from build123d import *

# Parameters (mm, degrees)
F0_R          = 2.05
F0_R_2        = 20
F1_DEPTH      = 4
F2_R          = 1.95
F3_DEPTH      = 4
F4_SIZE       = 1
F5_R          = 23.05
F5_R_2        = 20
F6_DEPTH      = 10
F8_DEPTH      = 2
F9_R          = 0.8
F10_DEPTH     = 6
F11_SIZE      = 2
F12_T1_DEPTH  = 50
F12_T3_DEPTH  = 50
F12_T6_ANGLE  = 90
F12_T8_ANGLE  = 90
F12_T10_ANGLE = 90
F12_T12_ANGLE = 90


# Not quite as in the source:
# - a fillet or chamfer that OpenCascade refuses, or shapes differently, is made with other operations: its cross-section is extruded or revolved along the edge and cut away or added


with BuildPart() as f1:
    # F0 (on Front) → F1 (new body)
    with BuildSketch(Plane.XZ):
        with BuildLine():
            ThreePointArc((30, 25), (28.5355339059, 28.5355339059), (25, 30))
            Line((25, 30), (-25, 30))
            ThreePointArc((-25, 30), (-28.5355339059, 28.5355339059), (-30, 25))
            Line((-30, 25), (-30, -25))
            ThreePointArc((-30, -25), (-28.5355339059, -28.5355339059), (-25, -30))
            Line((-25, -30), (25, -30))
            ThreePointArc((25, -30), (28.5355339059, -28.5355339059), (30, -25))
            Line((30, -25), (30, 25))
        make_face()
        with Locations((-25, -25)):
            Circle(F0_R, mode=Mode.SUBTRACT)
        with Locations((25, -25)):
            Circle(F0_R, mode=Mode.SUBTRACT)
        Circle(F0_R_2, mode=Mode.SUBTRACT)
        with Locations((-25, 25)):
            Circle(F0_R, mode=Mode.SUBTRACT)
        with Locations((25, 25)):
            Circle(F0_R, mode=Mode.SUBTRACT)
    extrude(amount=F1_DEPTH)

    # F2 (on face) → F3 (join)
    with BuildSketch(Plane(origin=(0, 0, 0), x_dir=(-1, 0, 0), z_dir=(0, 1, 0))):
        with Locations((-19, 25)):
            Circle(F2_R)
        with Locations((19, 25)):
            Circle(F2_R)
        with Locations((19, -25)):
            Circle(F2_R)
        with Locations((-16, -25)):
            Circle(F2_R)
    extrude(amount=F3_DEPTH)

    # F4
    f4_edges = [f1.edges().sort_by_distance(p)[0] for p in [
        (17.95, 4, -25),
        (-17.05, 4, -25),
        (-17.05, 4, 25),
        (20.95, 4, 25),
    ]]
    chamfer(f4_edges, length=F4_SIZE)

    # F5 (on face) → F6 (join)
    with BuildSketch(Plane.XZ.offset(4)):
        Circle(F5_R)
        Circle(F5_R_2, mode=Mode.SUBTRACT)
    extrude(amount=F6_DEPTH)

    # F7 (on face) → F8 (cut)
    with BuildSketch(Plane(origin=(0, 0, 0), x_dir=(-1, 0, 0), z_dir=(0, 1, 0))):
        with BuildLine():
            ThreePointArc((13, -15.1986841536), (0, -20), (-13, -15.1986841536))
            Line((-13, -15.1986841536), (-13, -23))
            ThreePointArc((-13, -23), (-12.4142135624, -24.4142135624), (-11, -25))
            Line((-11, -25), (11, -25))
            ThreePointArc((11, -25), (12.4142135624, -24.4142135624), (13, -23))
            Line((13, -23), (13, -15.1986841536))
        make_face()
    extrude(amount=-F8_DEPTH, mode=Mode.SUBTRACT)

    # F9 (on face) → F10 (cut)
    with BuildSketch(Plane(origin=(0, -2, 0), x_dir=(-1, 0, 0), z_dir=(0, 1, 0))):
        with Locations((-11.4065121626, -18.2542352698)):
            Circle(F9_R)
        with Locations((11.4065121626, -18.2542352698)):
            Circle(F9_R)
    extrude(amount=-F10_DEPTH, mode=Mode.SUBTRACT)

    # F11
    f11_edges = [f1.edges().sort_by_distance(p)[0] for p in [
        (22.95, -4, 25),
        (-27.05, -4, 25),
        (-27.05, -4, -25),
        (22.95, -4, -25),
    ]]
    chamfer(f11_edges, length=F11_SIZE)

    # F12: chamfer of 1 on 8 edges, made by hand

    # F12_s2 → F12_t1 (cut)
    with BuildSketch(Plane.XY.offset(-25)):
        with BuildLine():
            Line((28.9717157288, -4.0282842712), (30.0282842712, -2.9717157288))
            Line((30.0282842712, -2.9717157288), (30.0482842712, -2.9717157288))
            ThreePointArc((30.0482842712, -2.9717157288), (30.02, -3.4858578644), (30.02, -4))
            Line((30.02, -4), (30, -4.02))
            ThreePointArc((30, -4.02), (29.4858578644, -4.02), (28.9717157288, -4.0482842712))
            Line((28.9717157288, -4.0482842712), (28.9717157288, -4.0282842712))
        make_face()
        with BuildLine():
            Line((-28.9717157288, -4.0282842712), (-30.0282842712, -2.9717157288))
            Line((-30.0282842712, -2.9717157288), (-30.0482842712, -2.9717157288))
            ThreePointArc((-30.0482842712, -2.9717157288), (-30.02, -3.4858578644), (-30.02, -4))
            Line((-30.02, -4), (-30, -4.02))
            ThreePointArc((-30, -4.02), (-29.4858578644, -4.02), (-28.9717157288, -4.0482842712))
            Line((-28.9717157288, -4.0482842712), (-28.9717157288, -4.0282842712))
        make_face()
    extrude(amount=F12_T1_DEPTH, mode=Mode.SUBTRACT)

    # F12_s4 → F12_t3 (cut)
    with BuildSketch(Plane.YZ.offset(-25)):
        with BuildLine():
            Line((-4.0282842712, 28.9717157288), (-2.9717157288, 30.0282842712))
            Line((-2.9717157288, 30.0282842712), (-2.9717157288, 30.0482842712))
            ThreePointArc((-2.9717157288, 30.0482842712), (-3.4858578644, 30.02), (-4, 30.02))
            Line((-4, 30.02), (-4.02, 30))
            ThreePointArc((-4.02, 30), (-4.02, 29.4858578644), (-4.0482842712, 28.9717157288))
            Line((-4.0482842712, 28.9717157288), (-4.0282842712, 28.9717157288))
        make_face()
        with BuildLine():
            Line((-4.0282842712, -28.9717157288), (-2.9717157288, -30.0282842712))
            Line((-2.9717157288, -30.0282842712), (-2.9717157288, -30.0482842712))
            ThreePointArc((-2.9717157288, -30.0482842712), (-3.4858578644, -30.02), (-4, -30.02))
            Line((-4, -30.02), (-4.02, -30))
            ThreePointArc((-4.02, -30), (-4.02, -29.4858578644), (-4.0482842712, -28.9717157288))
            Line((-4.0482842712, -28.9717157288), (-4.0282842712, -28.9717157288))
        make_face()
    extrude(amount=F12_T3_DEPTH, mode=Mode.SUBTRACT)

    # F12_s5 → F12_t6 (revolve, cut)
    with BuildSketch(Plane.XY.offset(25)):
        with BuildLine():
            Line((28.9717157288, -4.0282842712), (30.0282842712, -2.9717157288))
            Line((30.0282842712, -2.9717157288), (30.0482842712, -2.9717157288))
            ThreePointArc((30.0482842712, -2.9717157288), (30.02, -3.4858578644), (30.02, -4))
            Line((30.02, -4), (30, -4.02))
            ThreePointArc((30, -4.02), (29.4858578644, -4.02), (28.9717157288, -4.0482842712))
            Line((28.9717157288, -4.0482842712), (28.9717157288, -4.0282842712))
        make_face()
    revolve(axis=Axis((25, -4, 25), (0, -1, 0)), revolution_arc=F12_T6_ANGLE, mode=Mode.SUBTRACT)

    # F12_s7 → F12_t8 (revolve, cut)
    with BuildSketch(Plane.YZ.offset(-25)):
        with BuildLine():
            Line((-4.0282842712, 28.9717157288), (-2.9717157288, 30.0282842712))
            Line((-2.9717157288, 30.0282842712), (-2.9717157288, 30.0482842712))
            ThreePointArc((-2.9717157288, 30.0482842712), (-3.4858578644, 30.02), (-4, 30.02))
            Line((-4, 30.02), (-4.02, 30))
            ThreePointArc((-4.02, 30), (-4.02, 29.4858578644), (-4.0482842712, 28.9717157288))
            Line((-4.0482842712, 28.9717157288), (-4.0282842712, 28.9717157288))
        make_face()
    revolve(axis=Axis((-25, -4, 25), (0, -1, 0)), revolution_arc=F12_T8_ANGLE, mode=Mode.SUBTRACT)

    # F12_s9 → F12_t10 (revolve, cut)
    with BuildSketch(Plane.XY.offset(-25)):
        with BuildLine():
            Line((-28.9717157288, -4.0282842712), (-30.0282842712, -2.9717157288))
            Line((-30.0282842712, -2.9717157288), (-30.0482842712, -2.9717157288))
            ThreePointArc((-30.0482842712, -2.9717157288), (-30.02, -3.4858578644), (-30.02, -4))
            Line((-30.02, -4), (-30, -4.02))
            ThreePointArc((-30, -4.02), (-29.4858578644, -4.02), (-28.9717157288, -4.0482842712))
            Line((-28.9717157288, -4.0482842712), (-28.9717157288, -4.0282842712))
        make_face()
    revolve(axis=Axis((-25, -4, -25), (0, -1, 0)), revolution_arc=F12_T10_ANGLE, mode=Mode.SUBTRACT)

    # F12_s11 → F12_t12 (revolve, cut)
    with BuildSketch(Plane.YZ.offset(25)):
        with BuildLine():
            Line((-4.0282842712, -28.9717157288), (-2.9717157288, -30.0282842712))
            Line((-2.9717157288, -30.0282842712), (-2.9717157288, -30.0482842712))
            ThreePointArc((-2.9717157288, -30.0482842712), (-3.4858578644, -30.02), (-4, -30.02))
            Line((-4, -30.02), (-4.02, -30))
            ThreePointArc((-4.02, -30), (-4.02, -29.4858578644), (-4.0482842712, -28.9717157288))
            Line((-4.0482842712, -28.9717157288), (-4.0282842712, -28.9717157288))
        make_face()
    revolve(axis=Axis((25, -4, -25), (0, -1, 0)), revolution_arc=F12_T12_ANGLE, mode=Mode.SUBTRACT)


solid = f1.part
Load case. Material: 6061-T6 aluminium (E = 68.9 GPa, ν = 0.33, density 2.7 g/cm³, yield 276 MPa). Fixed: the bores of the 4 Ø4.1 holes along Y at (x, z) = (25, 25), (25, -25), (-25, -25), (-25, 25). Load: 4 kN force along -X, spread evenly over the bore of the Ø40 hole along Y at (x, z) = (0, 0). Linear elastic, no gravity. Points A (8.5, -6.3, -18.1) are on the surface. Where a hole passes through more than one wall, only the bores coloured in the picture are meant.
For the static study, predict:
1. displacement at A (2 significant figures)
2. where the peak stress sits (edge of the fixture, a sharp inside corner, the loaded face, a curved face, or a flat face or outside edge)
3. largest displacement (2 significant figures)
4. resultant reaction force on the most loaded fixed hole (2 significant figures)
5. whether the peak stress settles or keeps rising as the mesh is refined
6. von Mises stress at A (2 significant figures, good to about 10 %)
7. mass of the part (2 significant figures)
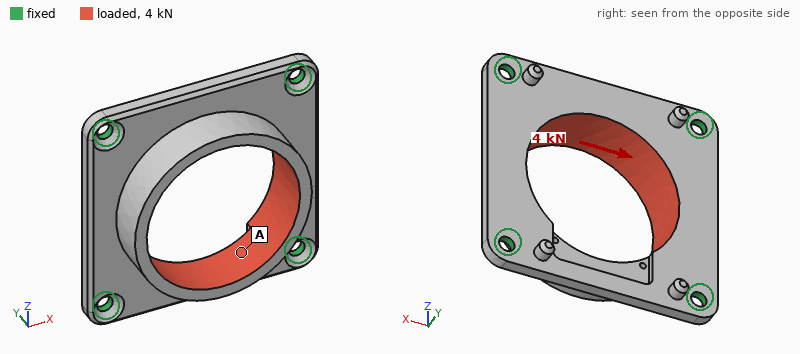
11 µm
edge of the fixture
35 µm
1.1 kN
keeps rising
25 MPa
34 g
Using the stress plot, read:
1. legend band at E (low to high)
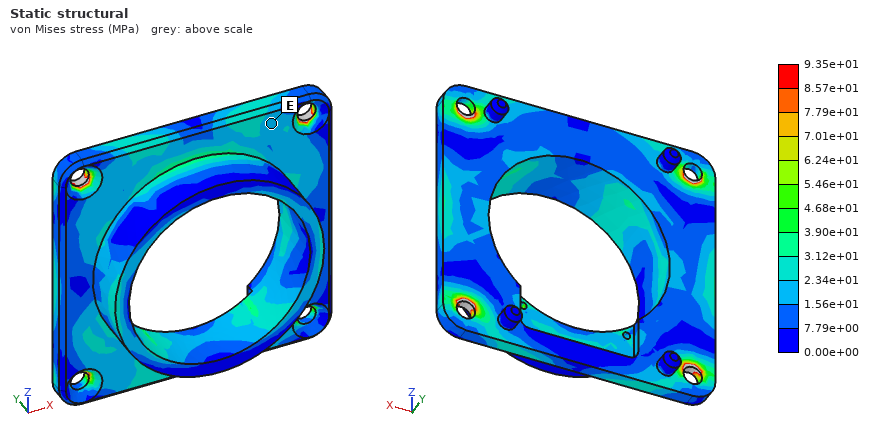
1.56e+01 to 2.34e+01 MPa
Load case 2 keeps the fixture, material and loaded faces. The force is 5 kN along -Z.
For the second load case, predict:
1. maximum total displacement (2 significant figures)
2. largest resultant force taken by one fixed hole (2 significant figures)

47 µm
1.4 kN
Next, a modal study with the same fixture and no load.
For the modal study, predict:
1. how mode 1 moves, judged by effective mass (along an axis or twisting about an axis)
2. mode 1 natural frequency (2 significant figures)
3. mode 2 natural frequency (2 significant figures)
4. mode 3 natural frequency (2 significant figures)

along Y
7200 Hz
8300 Hz
8400 Hz
